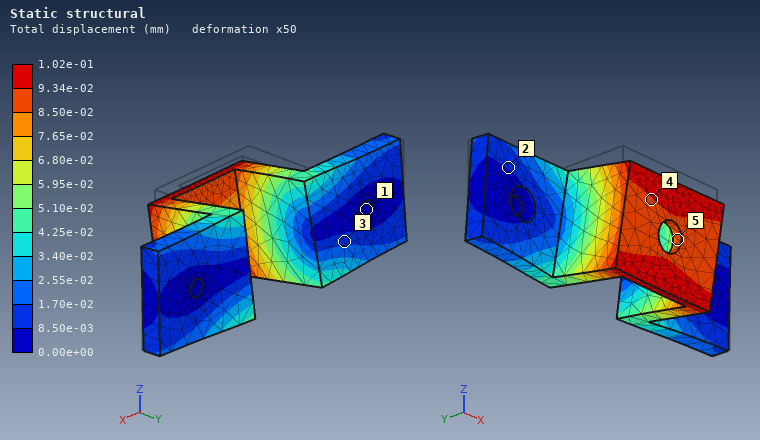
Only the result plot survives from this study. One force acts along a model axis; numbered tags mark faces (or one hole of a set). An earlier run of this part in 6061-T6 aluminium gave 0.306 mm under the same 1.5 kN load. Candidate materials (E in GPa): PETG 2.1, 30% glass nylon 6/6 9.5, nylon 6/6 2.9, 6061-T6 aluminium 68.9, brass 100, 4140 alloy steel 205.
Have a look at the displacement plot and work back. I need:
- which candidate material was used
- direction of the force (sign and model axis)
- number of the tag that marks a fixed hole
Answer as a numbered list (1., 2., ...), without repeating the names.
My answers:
1. 4140 alloy steel
2. -Z
3. 1
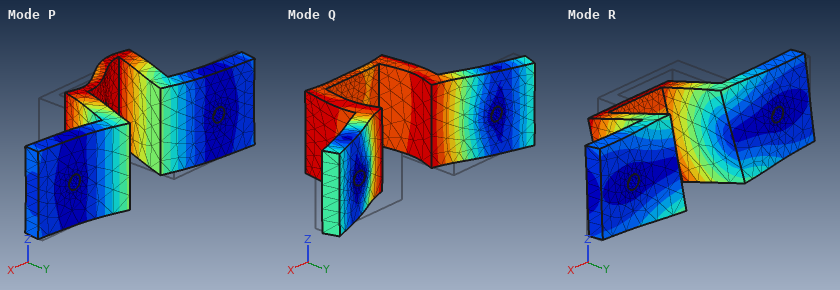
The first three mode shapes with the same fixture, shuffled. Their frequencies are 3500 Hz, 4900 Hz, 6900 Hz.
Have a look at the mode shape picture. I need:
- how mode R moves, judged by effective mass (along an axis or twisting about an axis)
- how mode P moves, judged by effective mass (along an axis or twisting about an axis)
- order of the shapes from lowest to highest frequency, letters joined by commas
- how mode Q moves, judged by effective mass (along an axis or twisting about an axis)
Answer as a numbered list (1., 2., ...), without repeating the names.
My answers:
1. along Z
2. along X
3. R, P, Q
4. along Y
